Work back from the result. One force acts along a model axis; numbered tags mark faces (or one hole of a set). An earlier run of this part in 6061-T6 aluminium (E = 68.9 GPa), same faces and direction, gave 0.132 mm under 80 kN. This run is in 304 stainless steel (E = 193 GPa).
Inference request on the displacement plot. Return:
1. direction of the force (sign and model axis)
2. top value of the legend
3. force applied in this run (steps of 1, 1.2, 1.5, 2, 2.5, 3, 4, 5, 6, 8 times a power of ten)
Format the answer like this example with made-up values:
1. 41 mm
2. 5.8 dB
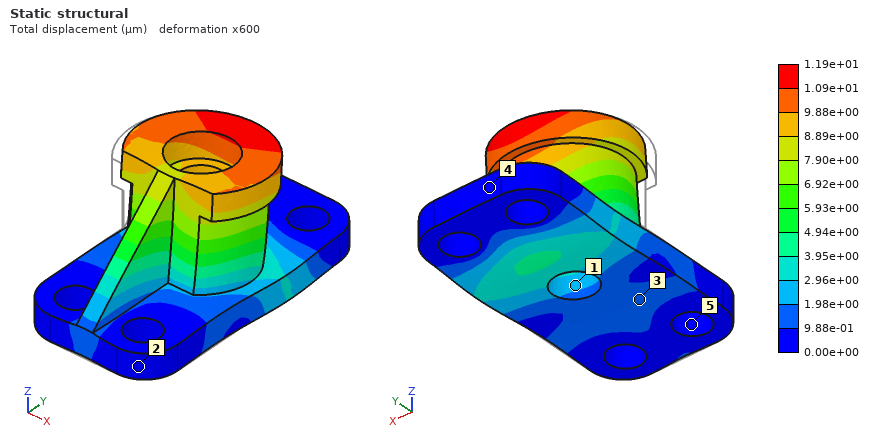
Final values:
1. +Y
2. 1.19e+01 µm
3. 20 kN
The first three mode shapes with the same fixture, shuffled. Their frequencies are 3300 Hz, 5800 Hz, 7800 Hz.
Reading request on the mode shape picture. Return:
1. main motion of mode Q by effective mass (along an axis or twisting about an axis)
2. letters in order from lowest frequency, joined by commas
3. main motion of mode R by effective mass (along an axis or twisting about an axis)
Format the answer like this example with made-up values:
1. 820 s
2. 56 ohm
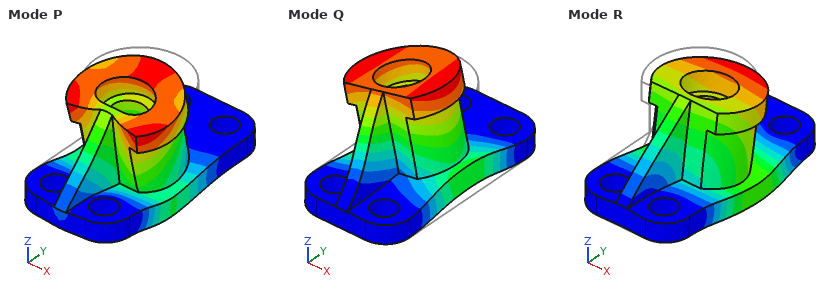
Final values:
1. along X
2. Q, R, P
3. along Z
